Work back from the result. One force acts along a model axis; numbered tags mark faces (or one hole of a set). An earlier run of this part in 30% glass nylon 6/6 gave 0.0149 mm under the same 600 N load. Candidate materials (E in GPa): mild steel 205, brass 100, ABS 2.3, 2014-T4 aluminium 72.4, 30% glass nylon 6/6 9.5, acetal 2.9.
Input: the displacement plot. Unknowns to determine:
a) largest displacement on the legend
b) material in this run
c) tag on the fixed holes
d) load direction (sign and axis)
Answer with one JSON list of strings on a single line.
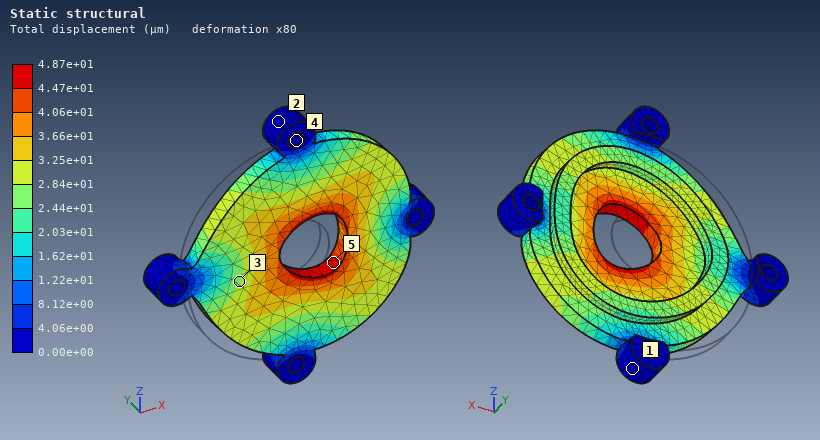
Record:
["4.87e+01 µm", "acetal", "4", "+X"]
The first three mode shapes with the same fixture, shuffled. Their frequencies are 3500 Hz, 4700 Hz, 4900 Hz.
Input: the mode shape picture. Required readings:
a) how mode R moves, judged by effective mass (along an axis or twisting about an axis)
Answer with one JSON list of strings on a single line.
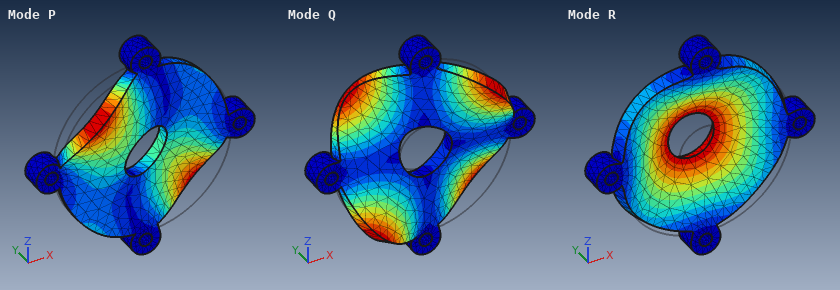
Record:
["along Y"]
